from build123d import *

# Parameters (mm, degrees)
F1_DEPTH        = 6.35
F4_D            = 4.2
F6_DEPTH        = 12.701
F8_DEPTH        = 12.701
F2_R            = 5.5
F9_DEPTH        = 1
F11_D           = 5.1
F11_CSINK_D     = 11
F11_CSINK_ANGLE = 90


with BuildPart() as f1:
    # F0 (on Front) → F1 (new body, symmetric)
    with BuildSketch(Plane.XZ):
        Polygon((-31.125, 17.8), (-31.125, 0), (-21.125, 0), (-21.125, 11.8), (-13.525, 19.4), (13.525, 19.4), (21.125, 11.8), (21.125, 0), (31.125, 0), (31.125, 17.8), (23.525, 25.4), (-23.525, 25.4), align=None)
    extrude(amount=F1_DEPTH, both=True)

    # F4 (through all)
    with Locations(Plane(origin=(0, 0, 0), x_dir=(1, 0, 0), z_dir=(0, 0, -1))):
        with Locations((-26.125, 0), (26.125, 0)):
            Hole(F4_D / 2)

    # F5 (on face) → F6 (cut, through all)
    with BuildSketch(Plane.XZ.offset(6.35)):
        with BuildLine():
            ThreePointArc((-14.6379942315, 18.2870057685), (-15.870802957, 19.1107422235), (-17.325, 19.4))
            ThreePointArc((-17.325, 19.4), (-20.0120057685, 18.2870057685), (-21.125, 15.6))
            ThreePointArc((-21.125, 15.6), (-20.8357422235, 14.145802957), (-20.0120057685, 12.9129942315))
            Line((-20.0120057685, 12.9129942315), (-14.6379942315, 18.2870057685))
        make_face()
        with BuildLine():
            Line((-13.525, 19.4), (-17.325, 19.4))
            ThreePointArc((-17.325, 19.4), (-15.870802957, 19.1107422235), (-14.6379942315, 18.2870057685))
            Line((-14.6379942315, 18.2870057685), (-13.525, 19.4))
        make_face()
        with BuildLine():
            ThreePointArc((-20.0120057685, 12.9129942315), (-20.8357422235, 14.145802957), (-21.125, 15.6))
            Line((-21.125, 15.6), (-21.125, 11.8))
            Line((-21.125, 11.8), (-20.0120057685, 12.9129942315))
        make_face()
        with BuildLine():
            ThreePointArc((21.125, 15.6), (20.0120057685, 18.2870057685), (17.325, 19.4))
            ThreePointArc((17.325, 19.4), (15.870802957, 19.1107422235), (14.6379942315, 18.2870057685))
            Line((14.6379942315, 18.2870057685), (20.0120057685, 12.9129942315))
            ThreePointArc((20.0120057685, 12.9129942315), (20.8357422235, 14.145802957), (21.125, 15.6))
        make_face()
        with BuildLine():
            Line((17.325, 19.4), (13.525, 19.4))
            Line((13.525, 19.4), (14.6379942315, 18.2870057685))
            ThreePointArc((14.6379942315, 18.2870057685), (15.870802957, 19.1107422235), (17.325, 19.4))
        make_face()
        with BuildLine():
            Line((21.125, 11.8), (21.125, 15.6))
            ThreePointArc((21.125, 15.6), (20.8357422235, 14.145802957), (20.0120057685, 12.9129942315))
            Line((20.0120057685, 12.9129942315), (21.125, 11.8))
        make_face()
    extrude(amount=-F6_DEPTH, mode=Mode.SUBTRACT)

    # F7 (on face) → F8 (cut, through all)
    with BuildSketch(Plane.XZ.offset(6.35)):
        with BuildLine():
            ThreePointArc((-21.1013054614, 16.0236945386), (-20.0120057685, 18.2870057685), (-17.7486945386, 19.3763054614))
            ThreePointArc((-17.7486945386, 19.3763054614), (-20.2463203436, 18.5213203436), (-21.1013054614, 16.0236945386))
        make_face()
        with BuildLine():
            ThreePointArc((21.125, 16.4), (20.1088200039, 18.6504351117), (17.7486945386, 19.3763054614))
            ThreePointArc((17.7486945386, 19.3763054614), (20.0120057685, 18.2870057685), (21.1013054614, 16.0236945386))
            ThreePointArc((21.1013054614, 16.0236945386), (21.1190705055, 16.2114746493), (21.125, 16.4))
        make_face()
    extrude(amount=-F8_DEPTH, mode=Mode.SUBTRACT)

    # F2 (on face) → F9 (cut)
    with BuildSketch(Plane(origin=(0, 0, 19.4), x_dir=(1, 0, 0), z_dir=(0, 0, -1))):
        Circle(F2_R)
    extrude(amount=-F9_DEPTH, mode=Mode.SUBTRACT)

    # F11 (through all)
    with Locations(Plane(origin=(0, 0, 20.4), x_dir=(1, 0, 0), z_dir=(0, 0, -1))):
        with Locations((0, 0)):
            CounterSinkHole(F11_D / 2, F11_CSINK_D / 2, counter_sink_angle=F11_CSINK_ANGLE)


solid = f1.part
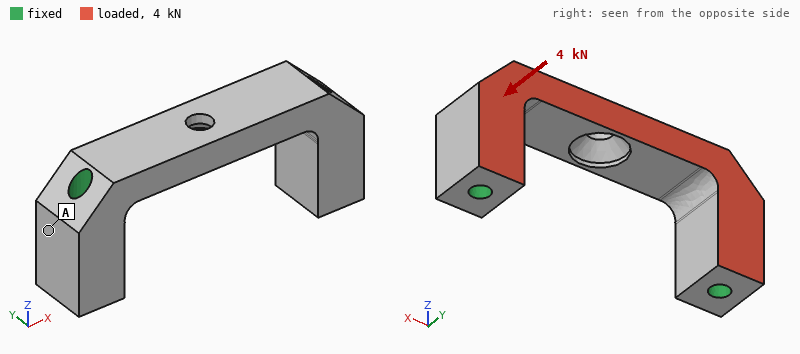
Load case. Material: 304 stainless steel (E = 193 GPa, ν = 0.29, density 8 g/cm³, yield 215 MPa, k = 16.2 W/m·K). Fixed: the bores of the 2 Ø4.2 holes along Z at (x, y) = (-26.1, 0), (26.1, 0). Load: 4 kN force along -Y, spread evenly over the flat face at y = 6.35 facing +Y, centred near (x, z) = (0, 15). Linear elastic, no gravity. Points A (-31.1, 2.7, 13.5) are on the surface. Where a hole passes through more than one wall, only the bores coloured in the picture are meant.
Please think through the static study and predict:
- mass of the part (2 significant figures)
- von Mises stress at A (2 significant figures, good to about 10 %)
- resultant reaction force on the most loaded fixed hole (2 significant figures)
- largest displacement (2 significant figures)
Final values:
64 g
7.6 MPa
2.0 kN
7.6 µm
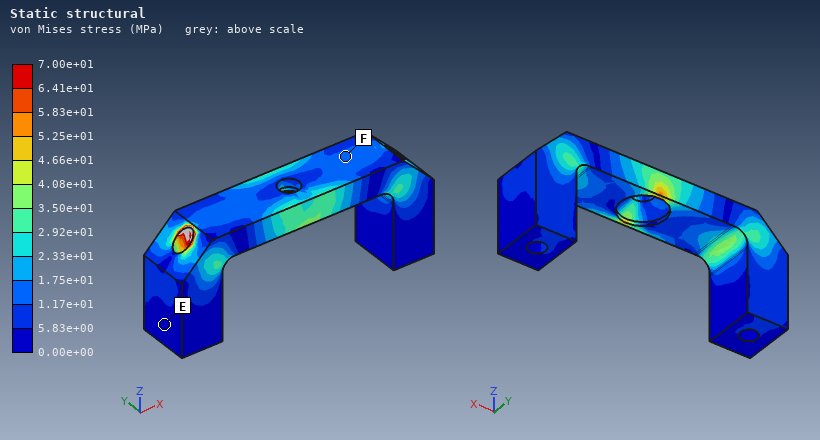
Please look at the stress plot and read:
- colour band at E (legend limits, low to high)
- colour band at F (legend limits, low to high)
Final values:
0.00e+00 to 5.83e+00 MPa
1.17e+01 to 1.75e+01 MPa
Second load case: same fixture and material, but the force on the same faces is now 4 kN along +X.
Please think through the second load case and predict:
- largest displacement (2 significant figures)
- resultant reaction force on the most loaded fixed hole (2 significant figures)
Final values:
1.8 µm
2.0 kN
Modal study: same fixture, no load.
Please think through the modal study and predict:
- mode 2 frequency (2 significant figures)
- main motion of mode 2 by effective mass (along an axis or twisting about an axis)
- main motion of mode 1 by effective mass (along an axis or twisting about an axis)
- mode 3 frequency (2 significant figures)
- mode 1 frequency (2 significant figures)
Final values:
17 kHz
along Y
along Z
27 kHz
13 kHz
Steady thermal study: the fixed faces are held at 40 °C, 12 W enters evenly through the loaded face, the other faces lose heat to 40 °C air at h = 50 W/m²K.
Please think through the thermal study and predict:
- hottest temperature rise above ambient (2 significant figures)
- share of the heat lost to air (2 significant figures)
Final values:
27 K
9.7 %
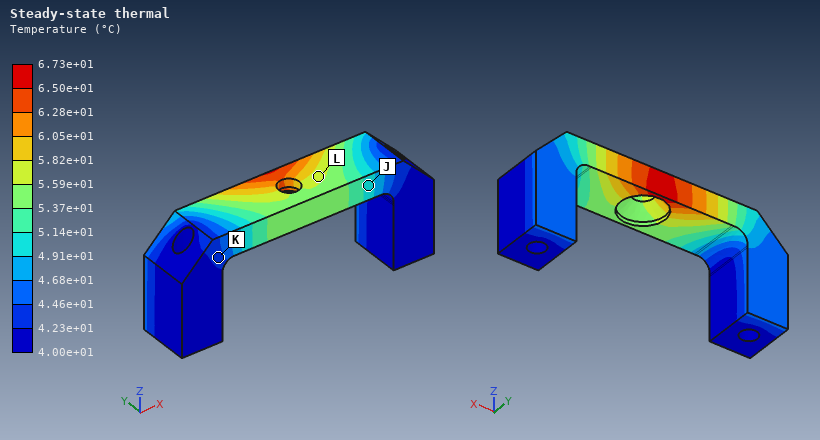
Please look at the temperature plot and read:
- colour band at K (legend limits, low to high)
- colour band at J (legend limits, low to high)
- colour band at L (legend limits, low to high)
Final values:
4.23e+01 to 4.46e+01 °C
4.91e+01 to 5.14e+01 °C
5.59e+01 to 5.82e+01 °C
